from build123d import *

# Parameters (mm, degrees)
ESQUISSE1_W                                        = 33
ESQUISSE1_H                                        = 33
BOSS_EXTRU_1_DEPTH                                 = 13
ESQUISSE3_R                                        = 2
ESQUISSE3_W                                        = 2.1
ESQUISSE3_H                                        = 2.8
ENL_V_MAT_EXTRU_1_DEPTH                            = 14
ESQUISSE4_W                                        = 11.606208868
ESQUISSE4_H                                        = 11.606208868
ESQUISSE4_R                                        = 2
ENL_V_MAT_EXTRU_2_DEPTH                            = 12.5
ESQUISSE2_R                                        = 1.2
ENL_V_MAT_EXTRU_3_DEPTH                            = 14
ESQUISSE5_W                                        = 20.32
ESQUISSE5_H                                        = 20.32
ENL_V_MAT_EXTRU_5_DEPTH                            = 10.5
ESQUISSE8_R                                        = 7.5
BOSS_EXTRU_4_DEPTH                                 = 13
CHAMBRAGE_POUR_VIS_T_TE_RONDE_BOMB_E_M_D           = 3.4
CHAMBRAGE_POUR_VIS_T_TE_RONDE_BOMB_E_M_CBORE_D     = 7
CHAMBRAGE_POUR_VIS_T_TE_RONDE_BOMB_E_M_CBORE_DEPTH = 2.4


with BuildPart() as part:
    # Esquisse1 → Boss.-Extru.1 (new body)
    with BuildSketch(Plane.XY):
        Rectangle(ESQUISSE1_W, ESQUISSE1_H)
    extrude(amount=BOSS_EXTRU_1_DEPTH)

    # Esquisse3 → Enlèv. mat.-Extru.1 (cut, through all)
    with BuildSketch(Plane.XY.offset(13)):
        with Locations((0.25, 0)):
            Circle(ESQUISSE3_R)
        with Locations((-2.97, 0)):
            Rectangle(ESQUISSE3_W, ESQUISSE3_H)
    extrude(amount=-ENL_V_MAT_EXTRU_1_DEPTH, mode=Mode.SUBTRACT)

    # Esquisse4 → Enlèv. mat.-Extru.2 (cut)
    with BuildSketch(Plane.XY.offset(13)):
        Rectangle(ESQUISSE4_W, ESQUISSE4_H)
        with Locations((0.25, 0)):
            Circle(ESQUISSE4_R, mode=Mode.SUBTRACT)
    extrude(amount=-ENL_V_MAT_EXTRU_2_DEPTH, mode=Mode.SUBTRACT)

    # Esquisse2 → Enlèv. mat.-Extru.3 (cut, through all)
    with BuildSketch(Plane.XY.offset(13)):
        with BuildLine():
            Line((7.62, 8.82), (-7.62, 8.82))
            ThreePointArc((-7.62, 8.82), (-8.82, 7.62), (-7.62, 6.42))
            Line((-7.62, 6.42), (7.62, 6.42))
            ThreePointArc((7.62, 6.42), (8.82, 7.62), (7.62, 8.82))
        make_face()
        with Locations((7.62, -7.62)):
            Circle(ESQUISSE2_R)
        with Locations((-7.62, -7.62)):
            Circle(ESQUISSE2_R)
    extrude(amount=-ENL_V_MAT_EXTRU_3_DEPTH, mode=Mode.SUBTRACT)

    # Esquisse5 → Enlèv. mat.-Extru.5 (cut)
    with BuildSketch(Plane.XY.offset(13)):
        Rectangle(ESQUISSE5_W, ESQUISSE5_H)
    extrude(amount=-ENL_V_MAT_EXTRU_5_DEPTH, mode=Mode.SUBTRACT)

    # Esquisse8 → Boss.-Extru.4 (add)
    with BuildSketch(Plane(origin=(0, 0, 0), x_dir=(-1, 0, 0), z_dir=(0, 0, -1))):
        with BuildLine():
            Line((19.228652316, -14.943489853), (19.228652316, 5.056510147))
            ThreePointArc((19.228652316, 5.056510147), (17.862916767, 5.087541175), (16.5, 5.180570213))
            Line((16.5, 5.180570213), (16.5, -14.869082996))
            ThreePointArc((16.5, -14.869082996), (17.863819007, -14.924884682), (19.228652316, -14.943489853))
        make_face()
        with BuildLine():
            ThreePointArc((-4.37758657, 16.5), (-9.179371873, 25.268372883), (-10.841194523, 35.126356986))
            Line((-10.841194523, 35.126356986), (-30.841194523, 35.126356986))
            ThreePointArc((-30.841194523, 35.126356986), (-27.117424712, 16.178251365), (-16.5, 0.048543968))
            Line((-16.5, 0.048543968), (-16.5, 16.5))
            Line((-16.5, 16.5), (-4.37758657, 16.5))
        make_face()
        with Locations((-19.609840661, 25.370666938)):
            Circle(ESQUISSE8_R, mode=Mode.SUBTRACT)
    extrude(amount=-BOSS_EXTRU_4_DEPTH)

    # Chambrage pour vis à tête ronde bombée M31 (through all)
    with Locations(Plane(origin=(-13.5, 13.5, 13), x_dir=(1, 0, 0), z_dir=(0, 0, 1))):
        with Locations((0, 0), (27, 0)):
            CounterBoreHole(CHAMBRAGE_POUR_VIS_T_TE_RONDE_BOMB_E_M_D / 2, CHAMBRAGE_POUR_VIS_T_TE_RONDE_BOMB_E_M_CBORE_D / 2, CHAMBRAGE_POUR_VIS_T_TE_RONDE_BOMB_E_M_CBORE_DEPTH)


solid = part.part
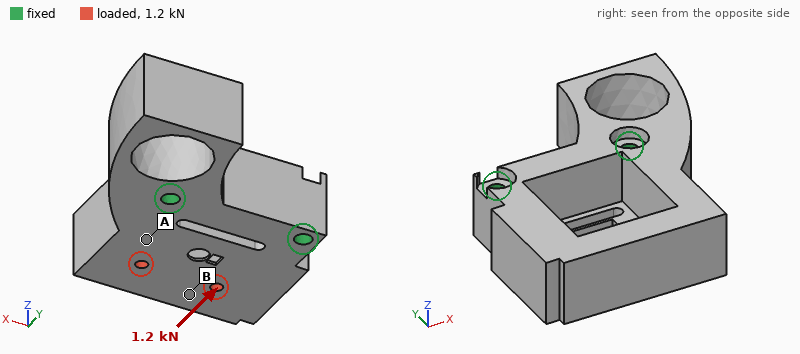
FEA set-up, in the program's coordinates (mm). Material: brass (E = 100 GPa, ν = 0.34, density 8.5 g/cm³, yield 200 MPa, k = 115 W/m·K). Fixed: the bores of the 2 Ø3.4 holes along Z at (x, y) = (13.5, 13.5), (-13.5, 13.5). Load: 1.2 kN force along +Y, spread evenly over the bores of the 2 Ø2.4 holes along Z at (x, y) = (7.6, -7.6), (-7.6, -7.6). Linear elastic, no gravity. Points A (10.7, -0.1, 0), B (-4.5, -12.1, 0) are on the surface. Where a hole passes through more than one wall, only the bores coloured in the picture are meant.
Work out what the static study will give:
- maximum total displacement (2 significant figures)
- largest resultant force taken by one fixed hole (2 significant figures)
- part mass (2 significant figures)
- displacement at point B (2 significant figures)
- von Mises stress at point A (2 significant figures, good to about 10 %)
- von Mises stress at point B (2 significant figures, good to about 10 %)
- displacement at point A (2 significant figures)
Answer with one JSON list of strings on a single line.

["9.2 µm", "620 N", "120 g", "7.5 µm", "19 MPa", "4.4 MPa", "3.3 µm"]
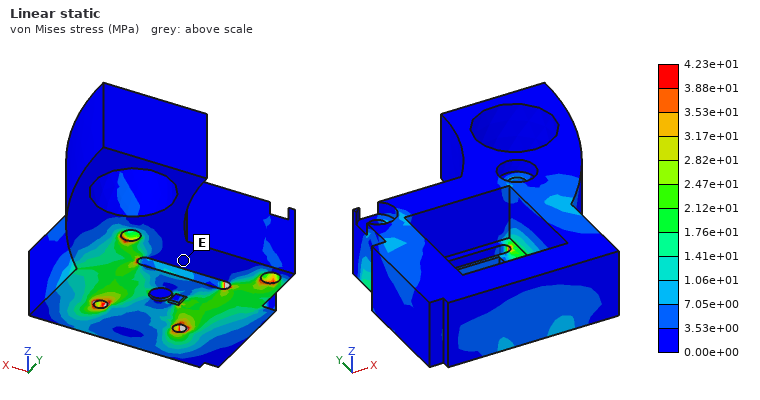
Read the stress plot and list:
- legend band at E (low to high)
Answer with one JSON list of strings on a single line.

["0.00e+00 to 3.53e+00 MPa"]
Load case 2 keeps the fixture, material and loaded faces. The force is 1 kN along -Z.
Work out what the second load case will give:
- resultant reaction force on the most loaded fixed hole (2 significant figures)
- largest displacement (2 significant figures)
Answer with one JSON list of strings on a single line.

["510 N", "27 µm"]
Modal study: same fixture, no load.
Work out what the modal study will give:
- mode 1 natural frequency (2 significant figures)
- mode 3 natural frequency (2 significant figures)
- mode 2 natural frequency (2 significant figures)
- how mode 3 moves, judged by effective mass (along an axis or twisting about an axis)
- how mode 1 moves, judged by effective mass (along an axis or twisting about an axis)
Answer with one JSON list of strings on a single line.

["4800 Hz", "7200 Hz", "5700 Hz", "along X", "along Z"]
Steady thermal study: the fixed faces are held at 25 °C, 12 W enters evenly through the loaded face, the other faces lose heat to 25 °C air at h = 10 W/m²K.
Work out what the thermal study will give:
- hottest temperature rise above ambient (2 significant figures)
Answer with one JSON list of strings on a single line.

["17 K"]
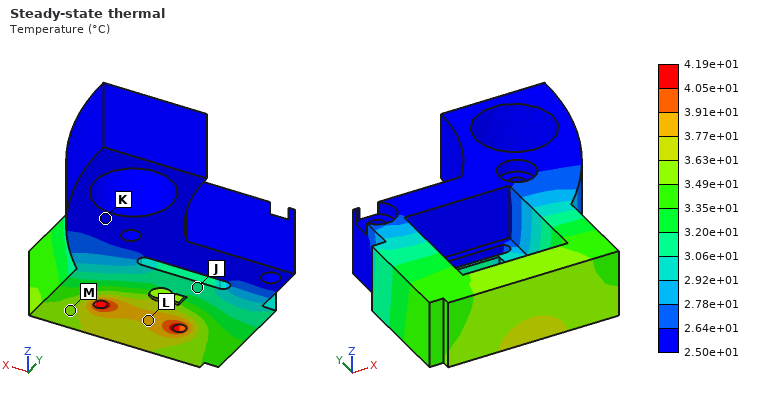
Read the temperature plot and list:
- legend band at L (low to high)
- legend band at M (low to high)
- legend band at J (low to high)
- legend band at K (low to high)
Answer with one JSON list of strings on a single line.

["3.77e+01 to 3.91e+01 °C", "3.49e+01 to 3.63e+01 °C", "3.06e+01 to 3.20e+01 °C", "2.50e+01 to 2.64e+01 °C"]
